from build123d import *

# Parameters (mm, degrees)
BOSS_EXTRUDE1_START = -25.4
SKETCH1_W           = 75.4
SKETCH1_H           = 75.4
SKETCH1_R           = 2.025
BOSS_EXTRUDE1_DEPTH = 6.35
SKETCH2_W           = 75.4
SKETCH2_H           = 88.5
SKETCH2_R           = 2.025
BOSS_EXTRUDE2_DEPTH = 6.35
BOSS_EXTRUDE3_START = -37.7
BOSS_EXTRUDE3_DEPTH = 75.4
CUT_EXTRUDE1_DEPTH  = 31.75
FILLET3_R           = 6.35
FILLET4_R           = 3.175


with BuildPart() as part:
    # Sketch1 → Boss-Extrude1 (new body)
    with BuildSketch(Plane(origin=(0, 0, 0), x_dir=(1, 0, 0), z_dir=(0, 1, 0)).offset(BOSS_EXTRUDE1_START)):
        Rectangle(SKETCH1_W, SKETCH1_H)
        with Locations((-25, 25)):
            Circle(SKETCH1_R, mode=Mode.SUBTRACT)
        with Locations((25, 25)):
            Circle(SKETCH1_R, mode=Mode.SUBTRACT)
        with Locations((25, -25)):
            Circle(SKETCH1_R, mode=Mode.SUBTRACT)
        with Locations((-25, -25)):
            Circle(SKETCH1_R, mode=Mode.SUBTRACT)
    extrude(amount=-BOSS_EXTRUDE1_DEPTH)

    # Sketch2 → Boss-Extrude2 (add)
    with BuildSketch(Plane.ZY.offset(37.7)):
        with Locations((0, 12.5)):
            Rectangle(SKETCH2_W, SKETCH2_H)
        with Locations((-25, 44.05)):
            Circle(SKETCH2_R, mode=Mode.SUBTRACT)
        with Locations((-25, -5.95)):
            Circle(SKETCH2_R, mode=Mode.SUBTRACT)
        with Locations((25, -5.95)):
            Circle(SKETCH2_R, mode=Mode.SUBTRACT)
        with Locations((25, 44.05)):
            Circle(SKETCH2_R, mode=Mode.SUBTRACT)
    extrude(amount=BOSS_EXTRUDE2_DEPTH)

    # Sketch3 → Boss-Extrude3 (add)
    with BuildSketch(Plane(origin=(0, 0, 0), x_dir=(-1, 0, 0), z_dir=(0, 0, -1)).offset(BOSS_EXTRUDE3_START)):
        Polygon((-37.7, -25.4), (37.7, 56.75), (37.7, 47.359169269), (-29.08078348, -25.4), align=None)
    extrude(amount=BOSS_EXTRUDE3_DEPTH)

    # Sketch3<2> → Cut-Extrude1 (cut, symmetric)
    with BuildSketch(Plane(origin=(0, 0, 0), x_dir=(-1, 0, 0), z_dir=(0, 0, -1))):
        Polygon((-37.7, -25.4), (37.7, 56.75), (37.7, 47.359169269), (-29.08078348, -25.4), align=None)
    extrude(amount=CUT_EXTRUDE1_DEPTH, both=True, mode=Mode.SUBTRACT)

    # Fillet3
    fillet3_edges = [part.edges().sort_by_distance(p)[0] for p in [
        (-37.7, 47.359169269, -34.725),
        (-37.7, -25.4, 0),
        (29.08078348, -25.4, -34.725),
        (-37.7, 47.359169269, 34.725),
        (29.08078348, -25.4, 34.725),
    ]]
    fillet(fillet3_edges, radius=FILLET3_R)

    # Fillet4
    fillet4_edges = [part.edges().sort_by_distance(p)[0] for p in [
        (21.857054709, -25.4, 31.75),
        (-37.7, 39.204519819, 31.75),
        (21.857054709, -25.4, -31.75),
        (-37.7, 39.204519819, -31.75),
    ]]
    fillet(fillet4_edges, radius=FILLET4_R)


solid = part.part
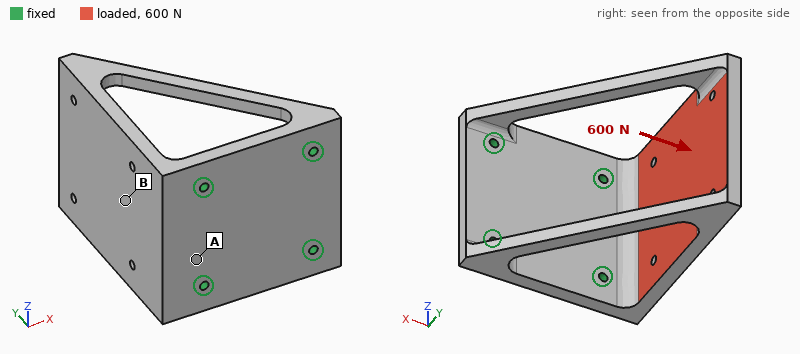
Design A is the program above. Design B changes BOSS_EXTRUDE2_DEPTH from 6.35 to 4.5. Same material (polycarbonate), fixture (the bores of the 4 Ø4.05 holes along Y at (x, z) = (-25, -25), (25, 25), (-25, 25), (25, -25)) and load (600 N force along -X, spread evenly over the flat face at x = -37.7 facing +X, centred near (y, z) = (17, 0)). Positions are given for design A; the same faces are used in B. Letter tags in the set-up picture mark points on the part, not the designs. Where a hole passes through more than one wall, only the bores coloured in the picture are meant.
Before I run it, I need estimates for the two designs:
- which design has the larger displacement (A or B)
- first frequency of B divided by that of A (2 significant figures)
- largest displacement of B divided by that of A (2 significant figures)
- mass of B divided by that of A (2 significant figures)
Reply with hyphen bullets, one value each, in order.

- B
- 1.0
- 1.5
- 0.86
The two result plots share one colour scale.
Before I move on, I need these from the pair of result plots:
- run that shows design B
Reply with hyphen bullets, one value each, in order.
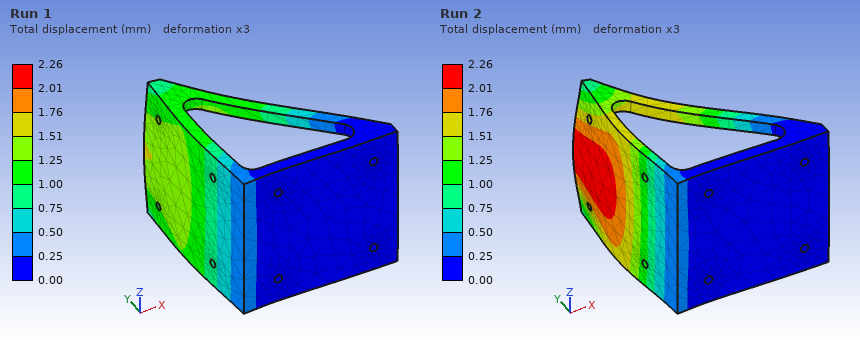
- Run 2
